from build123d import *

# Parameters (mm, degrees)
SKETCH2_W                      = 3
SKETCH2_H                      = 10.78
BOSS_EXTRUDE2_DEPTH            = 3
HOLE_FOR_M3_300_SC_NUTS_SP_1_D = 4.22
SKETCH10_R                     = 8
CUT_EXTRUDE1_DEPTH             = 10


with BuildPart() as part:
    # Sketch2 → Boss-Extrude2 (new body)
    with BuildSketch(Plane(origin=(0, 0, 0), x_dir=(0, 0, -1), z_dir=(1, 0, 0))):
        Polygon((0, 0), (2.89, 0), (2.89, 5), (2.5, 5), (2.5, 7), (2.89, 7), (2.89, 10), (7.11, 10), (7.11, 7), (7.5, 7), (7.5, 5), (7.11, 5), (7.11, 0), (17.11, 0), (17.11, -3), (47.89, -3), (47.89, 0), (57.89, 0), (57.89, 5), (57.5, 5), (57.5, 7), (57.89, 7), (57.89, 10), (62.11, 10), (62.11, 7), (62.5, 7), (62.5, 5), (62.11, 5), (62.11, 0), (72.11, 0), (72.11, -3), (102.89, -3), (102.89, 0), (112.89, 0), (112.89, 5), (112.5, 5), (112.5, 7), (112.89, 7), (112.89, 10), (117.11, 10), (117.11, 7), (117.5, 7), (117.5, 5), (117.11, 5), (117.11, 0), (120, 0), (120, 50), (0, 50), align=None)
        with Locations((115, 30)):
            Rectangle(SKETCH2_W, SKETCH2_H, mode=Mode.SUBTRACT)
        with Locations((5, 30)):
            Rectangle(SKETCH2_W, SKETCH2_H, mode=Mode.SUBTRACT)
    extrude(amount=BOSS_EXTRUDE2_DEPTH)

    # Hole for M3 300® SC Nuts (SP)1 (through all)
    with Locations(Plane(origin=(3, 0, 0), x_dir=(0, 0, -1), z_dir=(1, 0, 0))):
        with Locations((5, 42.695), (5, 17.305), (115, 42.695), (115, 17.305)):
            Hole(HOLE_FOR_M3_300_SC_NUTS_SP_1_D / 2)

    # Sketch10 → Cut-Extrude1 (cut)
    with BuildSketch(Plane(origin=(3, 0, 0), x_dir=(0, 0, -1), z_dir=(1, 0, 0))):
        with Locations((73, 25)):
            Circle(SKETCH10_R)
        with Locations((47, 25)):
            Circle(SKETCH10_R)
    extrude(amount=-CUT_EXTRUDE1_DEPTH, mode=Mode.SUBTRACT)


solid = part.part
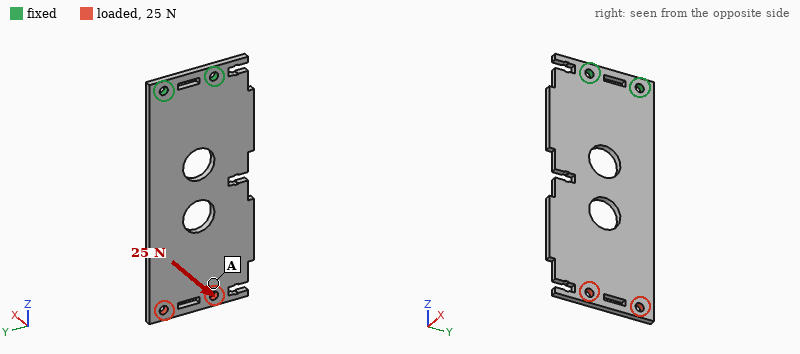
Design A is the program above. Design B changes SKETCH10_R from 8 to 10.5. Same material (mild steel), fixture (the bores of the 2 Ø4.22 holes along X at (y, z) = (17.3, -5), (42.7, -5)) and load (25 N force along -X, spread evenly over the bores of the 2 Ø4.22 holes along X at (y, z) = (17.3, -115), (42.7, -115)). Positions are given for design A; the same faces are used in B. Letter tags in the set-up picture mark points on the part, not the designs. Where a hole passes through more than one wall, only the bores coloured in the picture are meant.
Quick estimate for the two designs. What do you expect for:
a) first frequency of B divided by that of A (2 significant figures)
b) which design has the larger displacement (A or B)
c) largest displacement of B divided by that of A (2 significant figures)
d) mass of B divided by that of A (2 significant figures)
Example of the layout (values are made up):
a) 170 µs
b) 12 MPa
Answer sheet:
a) 0.98
b) B
c) 1.1
d) 0.95
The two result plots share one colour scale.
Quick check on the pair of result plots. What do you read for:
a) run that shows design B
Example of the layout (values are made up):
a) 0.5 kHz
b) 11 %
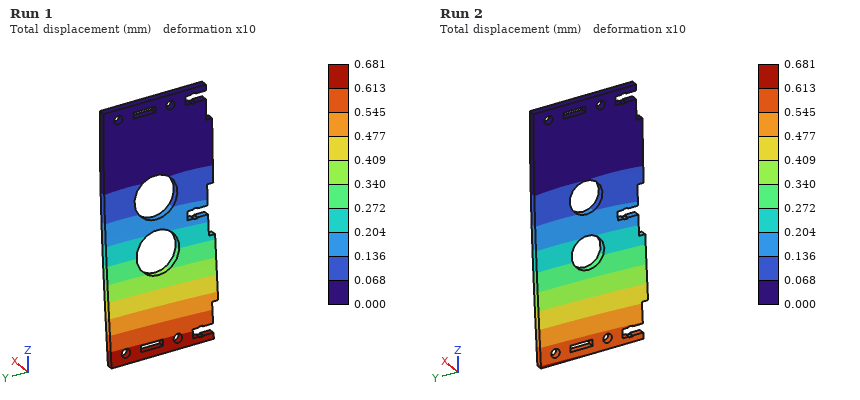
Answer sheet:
a) Run 1
